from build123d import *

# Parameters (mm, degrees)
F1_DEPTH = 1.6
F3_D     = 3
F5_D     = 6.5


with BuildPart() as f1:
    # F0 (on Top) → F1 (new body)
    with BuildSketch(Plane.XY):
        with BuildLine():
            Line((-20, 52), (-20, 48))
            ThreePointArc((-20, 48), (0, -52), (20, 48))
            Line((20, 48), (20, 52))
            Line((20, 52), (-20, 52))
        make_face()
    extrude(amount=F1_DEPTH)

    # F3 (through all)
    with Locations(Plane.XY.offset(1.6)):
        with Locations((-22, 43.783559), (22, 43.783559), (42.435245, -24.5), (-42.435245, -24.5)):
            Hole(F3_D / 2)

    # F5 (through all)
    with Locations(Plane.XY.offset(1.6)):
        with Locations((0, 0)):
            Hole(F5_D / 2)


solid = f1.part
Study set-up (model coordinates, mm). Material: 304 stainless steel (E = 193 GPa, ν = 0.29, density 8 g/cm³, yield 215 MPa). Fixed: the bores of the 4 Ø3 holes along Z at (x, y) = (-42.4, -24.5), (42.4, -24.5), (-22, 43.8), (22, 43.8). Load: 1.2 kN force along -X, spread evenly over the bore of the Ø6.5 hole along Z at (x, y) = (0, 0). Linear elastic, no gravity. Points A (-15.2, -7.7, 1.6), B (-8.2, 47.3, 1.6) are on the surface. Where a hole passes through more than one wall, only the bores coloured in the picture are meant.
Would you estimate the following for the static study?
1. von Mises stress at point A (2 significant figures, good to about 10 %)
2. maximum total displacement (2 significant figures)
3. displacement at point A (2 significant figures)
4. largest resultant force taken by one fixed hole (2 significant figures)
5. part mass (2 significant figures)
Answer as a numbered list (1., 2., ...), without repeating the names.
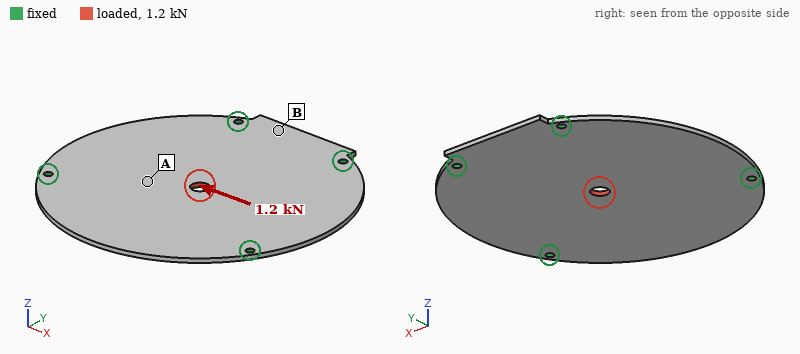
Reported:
1. 14 MPa
2. 4.3 µm
3. 2.5 µm
4. 380 N
5. 110 g
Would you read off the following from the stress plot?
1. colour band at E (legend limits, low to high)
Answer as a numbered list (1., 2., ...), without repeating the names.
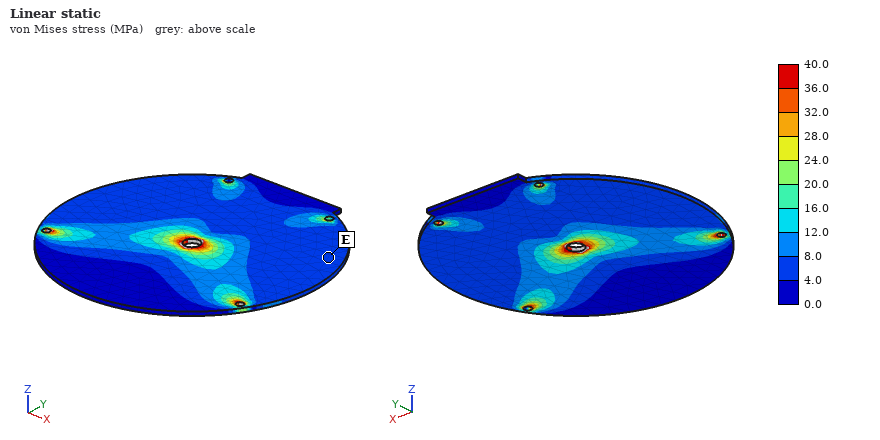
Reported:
1. 4.0 to 8.0 MPa
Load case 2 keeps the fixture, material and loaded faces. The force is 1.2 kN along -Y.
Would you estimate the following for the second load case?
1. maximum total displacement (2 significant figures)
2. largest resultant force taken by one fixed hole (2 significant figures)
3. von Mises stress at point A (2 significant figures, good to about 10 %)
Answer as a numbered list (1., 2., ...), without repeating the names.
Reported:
1. 4.3 µm
2. 340 N
3. 8.3 MPa
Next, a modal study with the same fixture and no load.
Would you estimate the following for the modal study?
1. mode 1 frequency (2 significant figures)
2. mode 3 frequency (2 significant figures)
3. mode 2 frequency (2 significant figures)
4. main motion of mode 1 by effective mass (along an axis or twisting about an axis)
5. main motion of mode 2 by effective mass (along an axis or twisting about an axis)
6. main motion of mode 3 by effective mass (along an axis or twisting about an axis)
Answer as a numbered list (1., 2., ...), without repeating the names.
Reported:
1. 840 Hz
2. 1400 Hz
3. 1100 Hz
4. along Z
5. along Z
6. twisting about Y
